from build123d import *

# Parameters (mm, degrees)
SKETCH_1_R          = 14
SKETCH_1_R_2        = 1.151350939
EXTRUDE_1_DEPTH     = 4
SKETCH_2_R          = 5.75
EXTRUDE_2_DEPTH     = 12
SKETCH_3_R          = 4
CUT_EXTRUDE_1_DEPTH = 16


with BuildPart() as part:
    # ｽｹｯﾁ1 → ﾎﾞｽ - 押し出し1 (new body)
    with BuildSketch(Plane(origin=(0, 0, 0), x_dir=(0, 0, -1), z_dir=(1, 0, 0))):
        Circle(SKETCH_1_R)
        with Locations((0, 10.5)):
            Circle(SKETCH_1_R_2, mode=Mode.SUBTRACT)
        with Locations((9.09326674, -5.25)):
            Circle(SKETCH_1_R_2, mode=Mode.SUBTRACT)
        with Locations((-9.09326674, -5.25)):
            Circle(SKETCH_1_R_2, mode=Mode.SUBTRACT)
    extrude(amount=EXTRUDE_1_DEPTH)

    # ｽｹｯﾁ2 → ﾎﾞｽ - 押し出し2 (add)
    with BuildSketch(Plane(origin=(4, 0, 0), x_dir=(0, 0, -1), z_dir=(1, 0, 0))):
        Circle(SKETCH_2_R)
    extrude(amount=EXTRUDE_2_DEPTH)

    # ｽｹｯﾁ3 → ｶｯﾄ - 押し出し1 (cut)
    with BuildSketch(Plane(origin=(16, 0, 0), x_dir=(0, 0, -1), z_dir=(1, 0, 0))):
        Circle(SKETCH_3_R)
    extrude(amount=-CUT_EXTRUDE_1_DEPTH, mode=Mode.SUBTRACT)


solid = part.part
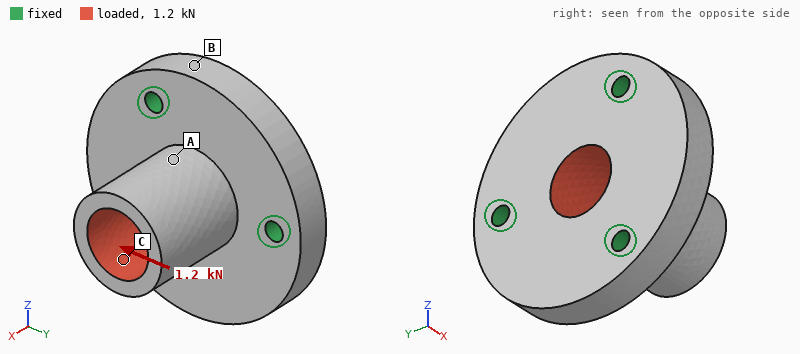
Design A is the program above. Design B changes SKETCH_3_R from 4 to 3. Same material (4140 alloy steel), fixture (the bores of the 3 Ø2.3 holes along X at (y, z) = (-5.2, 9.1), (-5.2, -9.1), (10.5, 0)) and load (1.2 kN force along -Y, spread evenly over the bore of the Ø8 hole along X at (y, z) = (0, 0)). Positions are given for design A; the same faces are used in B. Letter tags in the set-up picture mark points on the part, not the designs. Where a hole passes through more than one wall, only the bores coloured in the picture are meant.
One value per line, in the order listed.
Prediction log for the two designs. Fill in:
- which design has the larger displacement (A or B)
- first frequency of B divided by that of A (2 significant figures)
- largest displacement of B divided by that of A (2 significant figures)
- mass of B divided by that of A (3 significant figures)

A
0.95
0.80
1.12
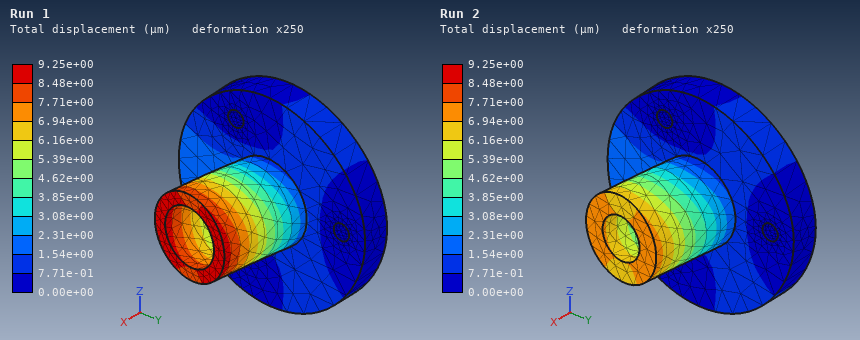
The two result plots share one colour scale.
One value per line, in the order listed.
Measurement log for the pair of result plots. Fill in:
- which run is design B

Run 2
